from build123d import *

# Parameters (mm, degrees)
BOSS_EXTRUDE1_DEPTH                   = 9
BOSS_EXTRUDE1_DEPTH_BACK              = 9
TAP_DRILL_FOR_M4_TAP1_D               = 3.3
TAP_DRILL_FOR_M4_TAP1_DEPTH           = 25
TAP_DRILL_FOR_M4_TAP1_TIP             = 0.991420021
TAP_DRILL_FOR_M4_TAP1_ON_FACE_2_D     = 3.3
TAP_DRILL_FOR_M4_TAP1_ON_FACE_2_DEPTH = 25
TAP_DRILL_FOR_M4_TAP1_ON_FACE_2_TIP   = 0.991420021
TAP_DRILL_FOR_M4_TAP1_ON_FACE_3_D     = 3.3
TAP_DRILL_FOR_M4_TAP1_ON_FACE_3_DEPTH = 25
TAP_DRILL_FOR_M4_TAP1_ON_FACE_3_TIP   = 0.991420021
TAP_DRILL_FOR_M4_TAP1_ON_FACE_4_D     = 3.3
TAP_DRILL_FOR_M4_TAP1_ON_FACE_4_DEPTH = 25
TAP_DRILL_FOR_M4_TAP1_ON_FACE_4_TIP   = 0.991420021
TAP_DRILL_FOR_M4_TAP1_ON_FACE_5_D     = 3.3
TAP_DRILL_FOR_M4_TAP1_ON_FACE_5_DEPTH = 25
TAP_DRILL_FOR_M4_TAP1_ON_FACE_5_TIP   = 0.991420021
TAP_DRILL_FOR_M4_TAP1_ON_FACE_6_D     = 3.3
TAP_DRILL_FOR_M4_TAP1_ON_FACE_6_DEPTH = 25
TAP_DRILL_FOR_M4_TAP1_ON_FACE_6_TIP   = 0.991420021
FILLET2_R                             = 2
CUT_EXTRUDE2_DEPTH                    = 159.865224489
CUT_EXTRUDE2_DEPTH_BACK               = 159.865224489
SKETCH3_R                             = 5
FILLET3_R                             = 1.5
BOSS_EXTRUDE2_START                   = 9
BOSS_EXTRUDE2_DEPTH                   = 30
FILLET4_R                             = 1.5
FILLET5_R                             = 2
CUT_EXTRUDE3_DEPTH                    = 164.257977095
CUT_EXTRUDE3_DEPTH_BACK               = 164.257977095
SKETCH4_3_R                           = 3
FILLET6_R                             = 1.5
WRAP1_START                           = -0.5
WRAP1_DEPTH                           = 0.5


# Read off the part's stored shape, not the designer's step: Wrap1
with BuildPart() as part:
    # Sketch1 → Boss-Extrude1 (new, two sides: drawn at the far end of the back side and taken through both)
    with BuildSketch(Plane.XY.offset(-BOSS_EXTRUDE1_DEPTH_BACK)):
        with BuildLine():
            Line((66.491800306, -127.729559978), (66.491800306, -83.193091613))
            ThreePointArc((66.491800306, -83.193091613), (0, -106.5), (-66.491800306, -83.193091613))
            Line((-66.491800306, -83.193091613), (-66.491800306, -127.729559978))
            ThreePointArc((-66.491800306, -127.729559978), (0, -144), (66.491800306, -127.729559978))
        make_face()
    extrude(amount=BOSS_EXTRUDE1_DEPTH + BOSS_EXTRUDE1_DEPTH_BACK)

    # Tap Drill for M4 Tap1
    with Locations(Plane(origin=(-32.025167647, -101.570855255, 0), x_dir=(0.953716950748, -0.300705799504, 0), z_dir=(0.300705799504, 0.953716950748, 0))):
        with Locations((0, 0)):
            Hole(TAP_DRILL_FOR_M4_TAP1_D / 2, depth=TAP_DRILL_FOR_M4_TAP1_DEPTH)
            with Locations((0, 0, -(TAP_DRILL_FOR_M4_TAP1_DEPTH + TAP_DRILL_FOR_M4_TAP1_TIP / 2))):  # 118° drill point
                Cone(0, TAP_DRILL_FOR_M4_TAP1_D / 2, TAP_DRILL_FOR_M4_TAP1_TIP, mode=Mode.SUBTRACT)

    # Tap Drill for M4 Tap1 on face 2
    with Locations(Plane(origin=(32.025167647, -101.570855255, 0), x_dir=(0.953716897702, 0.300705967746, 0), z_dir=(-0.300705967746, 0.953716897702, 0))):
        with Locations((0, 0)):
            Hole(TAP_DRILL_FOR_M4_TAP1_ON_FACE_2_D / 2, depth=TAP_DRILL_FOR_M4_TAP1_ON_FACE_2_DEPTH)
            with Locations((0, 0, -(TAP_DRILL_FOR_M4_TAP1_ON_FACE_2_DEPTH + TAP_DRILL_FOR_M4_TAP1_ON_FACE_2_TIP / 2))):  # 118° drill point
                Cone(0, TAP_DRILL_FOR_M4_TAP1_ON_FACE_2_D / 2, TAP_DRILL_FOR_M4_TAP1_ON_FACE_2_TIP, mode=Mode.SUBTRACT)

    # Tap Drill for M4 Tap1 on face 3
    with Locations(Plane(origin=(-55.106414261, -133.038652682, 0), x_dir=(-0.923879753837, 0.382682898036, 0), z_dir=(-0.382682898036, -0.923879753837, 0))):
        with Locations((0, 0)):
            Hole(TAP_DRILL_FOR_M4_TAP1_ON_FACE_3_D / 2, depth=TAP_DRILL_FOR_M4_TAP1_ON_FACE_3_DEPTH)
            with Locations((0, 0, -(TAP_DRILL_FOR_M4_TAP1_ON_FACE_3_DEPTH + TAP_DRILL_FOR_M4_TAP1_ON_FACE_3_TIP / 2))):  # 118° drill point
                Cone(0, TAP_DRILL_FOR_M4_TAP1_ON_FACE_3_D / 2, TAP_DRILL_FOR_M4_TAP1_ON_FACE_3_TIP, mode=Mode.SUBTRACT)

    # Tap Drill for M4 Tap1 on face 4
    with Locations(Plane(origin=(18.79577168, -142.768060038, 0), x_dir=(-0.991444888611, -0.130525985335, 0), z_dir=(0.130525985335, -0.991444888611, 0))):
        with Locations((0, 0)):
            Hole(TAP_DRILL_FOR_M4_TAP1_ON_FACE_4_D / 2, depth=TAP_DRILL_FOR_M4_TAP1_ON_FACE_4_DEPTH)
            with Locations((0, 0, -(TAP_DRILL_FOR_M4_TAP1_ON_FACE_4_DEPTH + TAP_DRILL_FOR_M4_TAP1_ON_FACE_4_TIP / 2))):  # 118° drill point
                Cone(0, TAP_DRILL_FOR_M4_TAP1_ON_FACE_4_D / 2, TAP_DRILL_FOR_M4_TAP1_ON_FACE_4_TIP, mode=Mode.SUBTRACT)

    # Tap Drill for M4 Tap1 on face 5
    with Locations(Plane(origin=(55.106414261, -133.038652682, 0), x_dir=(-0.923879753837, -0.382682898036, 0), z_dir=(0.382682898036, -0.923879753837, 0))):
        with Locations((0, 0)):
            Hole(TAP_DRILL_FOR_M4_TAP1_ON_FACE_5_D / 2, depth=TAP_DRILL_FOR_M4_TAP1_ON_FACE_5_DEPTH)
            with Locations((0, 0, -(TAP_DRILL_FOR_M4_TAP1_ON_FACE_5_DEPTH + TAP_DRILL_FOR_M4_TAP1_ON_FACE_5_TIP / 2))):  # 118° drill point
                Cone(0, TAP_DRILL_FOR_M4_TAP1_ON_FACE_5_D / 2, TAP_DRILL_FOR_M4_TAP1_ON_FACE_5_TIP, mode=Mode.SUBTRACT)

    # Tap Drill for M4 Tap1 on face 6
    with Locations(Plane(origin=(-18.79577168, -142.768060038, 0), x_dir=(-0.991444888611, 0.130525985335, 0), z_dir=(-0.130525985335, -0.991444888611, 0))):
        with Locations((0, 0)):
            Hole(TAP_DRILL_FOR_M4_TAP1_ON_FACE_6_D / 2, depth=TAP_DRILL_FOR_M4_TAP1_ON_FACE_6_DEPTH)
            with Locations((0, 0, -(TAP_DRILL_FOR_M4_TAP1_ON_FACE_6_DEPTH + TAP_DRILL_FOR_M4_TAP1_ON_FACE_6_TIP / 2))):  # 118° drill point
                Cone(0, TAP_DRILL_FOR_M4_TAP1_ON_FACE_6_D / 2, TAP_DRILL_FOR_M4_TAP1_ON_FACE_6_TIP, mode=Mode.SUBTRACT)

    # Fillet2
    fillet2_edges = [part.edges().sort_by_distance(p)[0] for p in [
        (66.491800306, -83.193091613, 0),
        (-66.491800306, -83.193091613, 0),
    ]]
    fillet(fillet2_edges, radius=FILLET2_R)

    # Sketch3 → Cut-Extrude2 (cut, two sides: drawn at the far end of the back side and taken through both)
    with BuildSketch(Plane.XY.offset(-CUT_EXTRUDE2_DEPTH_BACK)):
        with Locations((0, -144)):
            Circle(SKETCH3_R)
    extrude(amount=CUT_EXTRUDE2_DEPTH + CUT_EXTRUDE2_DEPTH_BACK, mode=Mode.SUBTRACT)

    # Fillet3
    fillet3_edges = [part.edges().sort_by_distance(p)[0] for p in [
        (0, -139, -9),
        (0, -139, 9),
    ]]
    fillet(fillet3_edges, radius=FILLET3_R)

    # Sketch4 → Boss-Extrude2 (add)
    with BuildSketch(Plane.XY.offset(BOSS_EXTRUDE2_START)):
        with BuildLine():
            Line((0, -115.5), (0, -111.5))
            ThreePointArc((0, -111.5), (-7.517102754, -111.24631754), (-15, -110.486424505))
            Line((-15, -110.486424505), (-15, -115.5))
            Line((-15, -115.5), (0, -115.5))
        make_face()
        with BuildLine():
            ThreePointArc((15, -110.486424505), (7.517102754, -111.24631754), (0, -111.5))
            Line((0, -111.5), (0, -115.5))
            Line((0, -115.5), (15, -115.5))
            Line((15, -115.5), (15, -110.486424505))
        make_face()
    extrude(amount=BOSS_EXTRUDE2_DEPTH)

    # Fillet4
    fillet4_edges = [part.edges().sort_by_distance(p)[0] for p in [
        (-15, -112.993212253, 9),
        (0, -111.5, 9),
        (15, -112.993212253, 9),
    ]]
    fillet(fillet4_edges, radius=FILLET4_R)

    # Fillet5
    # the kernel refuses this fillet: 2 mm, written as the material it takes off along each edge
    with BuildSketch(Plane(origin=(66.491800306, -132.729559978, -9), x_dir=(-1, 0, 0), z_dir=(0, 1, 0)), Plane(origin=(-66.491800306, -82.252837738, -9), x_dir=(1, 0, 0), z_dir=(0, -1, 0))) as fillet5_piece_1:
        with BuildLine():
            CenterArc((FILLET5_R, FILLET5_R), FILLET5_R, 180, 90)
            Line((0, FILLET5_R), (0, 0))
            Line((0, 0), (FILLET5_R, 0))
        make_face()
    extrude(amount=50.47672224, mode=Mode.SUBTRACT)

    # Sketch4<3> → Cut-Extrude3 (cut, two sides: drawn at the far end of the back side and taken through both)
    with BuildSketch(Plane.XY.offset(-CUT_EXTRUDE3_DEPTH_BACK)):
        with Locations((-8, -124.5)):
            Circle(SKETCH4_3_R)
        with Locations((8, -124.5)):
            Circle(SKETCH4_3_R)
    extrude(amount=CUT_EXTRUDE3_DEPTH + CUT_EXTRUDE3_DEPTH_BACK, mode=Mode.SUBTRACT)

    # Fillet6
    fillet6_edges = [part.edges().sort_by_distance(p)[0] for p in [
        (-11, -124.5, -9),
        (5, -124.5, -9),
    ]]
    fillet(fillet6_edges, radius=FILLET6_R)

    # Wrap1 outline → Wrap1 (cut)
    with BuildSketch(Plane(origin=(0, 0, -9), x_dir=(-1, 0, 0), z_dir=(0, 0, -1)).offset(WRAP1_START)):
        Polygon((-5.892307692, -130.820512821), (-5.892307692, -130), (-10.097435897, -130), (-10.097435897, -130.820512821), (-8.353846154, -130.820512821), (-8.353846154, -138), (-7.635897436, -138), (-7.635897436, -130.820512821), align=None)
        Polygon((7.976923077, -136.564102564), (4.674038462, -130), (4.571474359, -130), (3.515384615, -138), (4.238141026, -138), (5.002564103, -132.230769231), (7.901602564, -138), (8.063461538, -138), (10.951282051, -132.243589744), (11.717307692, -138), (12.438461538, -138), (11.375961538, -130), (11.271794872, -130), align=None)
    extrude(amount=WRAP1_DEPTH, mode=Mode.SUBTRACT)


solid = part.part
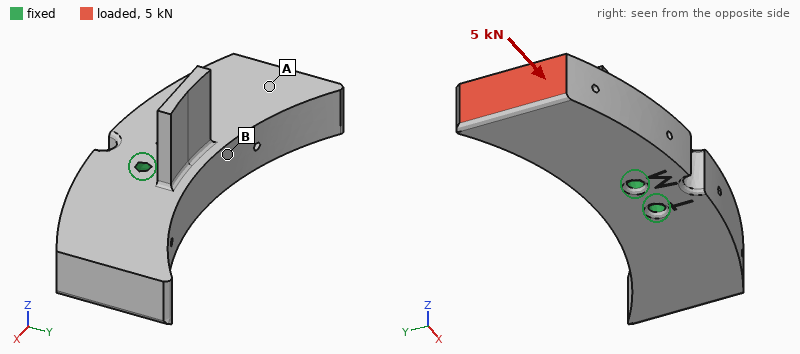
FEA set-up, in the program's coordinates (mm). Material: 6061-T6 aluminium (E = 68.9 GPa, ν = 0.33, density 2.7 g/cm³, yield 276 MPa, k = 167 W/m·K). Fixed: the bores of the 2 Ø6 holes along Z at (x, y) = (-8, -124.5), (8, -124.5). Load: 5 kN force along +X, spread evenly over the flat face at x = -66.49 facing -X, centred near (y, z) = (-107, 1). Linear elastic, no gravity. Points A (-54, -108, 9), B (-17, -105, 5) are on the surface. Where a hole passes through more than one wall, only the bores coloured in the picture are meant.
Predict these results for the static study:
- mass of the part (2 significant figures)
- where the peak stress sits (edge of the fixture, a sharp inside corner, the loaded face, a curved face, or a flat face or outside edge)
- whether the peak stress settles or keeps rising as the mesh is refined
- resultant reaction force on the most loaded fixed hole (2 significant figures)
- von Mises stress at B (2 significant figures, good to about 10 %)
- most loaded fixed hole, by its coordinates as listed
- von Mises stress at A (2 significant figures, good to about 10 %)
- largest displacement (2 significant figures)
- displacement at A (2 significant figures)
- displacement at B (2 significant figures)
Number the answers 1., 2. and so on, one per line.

1. 260 g
2. edge of the fixture
3. keeps rising
4. 5.0 kN
5. 29 MPa
6. (-8, -124.5)
7. 12 MPa
8. 68 µm
9. 41 µm
10. 14 µm
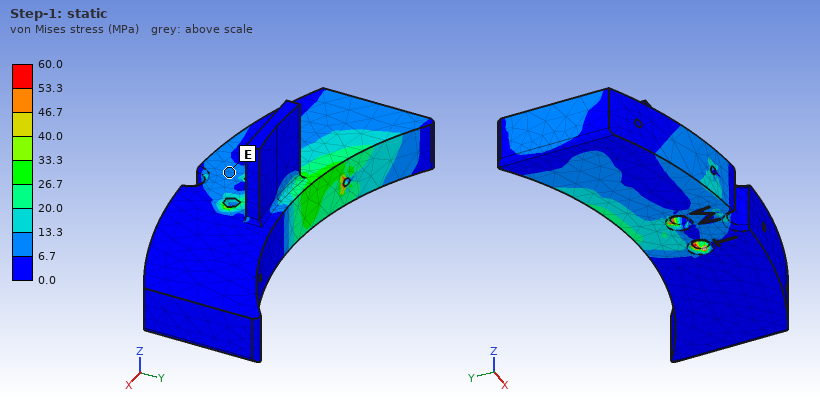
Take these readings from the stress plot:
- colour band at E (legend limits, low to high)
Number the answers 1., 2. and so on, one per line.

1. 6.7 to 13.3 MPa
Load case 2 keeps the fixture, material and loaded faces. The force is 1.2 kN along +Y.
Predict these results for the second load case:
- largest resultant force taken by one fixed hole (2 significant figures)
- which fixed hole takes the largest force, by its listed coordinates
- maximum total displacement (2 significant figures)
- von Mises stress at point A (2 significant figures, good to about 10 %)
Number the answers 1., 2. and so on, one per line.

1. 4.1 kN
2. (-8, -124.5)
3. 49 µm
4. 4.6 MPa
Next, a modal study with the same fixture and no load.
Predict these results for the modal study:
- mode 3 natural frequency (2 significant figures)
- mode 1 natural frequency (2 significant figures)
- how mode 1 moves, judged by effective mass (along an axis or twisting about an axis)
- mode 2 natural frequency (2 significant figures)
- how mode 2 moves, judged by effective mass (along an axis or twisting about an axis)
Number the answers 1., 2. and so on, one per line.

1. 3800 Hz
2. 3200 Hz
3. twisting about Y
4. 3400 Hz
5. along Z
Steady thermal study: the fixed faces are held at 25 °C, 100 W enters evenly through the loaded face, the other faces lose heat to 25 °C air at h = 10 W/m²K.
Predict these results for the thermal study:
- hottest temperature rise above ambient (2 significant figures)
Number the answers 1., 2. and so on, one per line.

1. 63 K
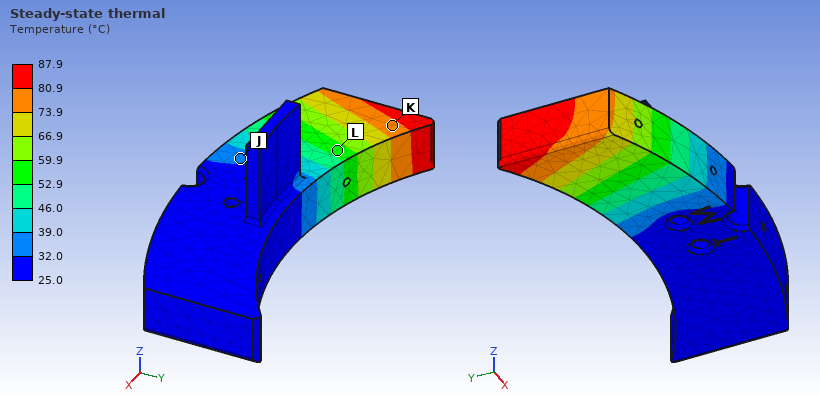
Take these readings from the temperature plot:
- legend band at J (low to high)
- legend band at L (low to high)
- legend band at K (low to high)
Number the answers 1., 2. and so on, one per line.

1. 32.0 to 39.0 °C
2. 52.9 to 59.9 °C
3. 73.9 to 80.9 °C
